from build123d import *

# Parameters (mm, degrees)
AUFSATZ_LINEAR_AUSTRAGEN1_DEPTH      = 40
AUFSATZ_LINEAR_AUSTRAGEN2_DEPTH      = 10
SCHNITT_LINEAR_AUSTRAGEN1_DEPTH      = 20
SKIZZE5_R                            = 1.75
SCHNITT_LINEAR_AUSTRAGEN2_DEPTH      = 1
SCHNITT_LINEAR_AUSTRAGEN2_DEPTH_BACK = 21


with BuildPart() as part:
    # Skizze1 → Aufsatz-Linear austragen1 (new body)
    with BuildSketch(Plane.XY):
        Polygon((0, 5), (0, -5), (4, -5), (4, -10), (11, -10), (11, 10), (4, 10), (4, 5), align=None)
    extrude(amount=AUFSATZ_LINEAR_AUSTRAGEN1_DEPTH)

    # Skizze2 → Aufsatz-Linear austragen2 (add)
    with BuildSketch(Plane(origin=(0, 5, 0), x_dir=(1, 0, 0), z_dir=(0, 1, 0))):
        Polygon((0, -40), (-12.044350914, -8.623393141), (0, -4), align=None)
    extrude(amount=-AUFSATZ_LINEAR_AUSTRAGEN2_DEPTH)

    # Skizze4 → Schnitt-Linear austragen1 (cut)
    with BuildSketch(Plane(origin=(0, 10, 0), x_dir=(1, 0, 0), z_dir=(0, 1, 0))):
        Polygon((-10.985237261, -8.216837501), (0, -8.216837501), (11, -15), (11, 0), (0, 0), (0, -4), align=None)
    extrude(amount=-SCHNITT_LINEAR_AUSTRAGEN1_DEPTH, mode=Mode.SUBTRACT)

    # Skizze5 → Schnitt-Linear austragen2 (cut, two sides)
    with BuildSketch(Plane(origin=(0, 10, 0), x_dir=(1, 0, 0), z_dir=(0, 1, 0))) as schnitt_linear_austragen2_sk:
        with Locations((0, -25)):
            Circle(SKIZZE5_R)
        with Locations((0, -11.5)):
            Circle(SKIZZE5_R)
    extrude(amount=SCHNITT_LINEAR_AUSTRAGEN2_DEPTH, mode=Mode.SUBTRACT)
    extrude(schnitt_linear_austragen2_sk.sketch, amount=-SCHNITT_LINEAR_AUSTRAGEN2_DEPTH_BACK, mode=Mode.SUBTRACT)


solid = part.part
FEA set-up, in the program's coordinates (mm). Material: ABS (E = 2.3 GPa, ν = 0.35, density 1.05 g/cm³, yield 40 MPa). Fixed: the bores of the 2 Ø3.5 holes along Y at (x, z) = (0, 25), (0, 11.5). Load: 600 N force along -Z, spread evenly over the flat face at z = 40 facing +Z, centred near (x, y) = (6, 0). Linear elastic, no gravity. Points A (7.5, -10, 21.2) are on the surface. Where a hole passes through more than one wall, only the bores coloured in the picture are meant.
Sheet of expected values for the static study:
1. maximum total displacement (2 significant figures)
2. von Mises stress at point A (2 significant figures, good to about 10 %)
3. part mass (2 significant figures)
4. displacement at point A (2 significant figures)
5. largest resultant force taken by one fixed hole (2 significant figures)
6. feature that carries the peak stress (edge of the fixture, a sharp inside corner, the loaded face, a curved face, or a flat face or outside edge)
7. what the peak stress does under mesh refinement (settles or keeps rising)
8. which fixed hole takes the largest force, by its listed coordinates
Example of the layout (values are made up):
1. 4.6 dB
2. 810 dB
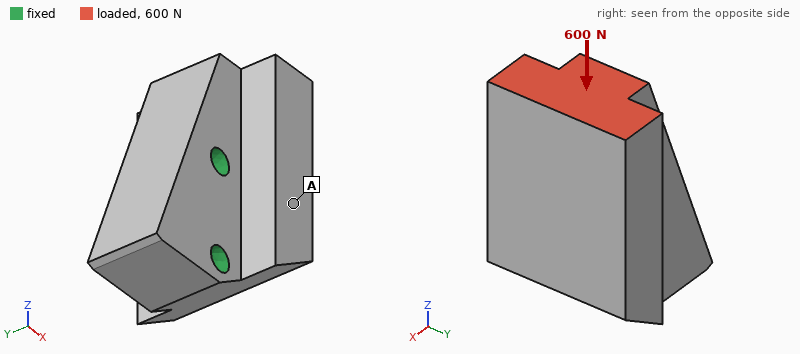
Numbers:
1. 83 µm
2. 1.9 MPa
3. 7.1 g
4. 27 µm
5. 460 N
6. edge of the fixture
7. keeps rising
8. (0, 25)
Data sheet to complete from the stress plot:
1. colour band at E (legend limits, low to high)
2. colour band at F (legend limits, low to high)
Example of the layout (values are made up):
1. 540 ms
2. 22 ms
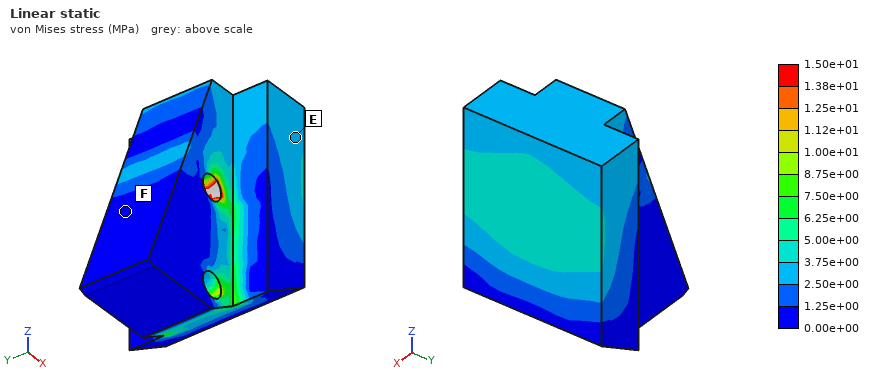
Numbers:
1. 2.50e+00 to 3.75e+00 MPa
2. 0.00e+00 to 1.25e+00 MPa
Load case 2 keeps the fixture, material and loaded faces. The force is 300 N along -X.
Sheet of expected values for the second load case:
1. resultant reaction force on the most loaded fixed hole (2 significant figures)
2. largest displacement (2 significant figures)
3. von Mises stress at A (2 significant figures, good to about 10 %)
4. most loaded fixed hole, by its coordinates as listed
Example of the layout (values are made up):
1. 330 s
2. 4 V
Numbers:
1. 560 N
2. 0.15 mm
3. 1.9 MPa
4. (0, 25)
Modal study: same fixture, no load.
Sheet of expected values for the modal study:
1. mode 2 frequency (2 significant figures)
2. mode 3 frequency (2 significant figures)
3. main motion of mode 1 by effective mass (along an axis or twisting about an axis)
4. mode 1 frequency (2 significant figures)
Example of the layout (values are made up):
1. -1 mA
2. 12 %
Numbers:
1. 7000 Hz
2. 8400 Hz
3. along Y
4. 5800 Hz
